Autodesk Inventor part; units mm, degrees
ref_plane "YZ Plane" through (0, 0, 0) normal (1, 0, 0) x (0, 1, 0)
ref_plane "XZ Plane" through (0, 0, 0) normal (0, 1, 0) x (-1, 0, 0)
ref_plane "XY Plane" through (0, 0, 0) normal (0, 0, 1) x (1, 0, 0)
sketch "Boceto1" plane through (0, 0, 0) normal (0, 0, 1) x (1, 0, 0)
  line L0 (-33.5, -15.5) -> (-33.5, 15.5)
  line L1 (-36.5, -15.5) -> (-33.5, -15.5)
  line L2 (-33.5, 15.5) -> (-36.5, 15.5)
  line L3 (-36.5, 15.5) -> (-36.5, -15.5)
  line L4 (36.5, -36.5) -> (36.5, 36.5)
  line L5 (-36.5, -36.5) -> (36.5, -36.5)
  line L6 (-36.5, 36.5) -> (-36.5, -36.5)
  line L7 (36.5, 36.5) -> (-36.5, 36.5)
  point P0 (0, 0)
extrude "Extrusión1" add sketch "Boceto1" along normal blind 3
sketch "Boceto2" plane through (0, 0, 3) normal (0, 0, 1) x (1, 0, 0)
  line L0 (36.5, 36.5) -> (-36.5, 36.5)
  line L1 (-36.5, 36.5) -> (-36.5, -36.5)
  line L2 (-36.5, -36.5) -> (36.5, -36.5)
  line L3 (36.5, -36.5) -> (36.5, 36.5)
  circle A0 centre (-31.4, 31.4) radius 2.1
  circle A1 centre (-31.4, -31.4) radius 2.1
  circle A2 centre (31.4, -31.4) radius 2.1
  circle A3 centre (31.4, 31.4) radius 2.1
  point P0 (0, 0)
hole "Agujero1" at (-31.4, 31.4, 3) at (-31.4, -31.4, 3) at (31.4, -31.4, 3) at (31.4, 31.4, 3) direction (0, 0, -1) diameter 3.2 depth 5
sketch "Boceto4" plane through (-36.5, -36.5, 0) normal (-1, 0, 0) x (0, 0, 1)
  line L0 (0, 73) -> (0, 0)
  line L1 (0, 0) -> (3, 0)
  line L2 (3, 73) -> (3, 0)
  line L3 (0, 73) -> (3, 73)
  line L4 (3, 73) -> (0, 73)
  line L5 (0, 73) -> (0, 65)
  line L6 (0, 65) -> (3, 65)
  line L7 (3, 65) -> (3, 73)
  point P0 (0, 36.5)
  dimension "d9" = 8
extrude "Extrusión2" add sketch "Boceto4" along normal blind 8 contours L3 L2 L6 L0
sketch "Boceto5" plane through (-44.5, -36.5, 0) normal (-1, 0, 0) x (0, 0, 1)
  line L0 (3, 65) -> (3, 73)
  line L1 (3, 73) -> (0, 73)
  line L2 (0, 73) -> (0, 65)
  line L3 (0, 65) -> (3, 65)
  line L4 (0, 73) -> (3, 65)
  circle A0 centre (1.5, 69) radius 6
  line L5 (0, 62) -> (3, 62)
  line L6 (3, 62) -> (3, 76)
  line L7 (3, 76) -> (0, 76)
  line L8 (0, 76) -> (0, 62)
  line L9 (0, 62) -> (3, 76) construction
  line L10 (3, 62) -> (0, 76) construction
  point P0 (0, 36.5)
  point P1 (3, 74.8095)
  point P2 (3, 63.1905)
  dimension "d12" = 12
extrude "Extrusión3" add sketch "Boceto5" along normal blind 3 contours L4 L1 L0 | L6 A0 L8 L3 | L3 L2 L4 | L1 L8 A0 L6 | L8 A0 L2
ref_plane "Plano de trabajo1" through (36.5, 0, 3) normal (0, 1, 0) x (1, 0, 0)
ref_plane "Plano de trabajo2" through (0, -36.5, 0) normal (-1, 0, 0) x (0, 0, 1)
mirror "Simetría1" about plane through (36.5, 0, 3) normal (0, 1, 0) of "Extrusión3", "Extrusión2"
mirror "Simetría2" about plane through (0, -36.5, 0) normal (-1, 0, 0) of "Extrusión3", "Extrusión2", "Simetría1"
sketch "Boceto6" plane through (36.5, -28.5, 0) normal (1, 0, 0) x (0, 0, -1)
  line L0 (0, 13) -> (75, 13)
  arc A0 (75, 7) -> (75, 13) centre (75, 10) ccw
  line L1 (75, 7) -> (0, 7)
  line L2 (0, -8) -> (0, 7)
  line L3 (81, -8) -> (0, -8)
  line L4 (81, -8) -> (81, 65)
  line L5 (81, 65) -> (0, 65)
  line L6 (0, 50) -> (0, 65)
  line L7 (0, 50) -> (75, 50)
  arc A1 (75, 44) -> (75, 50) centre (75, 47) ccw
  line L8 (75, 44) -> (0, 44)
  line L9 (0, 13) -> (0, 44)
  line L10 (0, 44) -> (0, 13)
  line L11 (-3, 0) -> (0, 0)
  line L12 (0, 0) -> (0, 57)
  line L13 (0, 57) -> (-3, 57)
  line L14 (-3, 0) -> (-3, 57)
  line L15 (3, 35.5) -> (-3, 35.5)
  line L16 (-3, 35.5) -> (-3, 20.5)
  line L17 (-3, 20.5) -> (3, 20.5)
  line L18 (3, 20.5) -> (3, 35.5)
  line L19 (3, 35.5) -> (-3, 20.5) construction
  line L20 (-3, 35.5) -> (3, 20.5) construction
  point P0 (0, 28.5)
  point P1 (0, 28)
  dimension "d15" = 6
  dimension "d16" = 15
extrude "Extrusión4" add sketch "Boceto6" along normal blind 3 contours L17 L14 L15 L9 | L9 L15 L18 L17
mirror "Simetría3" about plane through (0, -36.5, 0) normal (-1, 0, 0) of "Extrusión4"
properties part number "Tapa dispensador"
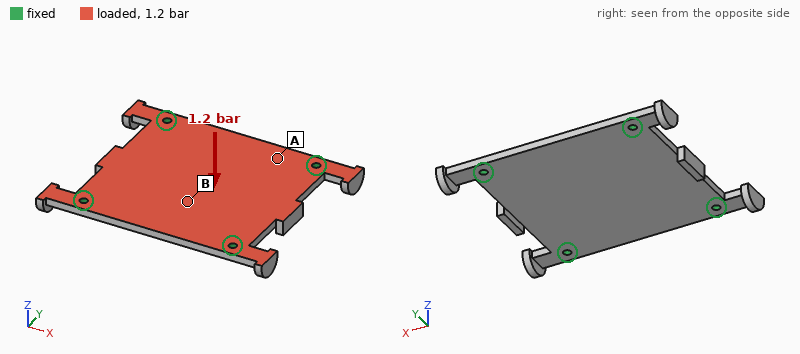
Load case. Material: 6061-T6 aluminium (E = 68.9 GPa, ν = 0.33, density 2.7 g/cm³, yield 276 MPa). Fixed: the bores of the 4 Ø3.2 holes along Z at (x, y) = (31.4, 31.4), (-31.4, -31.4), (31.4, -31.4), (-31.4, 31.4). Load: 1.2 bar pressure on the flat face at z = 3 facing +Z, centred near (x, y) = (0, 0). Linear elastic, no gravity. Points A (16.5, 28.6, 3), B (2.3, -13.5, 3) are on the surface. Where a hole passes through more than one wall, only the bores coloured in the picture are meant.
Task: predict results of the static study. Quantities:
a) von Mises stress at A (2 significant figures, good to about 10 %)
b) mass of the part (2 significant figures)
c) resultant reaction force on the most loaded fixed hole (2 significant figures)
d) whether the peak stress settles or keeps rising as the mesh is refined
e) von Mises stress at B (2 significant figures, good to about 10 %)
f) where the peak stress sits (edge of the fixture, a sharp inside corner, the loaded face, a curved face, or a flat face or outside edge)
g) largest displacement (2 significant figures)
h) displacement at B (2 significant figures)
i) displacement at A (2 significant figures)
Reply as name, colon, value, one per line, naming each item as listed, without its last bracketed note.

von Mises stress at A: 7.0 MPa
mass of the part: 49 g
resultant reaction force on the most loaded fixed hole: 170 N
whether the peak stress settles or keeps rising as the mesh is refined: keeps rising
von Mises stress at B: 16 MPa
where the peak stress sits: edge of the fixture
largest displacement: 86 µm
displacement at B: 76 µm
displacement at A: 31 µm
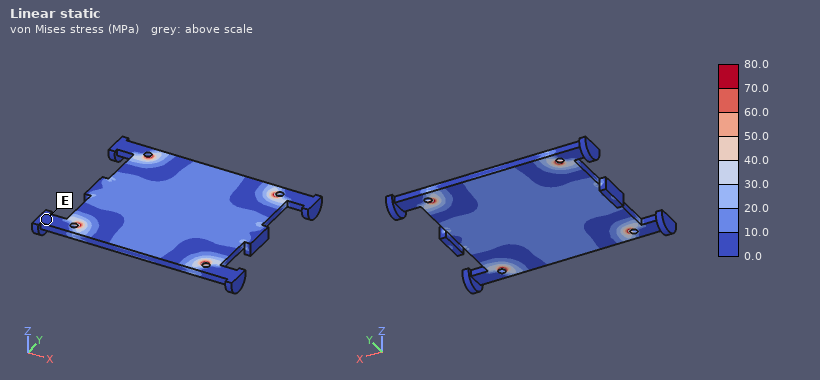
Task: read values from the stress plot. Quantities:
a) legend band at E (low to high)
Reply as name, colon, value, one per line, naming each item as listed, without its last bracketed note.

legend band at E: 0.0 to 10.0 MPa
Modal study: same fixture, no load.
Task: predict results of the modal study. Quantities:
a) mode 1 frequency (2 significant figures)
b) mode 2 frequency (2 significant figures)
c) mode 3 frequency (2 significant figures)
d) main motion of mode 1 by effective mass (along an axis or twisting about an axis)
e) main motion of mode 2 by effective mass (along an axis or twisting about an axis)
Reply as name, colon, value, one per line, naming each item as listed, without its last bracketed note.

mode 1 frequency: 2500 Hz
mode 2 frequency: 4000 Hz
mode 3 frequency: 4300 Hz
main motion of mode 1 by effective mass: along Z
main motion of mode 2 by effective mass: twisting about Y
